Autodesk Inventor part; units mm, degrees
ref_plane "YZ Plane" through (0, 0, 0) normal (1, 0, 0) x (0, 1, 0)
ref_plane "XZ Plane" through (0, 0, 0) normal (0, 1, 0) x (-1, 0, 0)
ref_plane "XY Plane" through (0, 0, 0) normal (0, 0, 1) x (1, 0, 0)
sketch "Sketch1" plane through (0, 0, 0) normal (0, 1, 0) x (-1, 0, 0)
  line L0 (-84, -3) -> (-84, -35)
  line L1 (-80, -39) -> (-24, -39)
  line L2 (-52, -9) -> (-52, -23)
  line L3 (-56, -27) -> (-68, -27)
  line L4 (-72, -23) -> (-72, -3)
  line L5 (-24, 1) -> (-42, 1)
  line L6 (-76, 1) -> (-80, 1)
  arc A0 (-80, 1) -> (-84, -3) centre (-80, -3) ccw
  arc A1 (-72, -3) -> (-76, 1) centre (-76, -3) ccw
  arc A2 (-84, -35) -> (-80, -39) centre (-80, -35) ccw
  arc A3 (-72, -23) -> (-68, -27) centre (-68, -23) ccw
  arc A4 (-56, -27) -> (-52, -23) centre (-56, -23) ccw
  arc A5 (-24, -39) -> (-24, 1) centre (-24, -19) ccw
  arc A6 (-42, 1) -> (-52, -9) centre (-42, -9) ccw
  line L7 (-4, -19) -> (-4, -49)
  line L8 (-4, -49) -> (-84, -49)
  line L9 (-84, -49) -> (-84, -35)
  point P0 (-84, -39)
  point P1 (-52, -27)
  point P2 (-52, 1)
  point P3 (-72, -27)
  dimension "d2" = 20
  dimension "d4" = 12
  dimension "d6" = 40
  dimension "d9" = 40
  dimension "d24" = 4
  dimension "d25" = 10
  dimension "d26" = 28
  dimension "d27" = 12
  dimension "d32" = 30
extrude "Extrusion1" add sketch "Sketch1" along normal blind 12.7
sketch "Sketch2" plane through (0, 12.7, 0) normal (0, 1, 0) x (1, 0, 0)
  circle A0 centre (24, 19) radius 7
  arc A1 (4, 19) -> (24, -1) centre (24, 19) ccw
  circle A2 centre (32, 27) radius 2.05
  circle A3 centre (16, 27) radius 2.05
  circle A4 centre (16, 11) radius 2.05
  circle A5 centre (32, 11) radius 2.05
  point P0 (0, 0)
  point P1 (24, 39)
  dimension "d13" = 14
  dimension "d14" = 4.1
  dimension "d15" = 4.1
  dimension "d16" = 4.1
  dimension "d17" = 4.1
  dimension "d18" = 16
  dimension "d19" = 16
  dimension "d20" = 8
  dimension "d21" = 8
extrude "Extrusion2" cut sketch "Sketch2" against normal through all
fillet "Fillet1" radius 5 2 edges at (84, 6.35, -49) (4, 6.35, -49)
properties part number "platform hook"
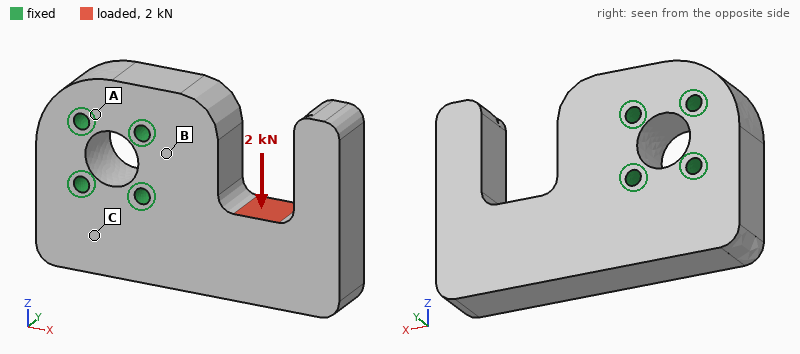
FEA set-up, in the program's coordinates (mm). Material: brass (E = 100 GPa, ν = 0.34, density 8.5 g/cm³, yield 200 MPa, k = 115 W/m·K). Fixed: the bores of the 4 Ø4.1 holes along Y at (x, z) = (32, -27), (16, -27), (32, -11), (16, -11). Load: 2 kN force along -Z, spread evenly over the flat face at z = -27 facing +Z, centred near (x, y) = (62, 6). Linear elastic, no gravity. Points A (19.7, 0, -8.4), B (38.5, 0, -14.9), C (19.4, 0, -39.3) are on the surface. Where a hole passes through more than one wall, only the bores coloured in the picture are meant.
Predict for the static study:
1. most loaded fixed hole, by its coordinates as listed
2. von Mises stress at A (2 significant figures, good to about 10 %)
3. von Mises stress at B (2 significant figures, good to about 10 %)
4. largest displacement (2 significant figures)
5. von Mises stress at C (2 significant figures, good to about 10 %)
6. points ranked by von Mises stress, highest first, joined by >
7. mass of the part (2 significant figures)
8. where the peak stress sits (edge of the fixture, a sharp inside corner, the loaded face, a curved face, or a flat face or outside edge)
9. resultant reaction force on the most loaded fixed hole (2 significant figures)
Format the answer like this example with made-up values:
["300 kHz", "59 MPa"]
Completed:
["(32, -11)", "4.1 MPa", "17 MPa", "26 µm", "7.9 MPa", "B > C > A", "340 g", "a curved face", "2.2 kN"]
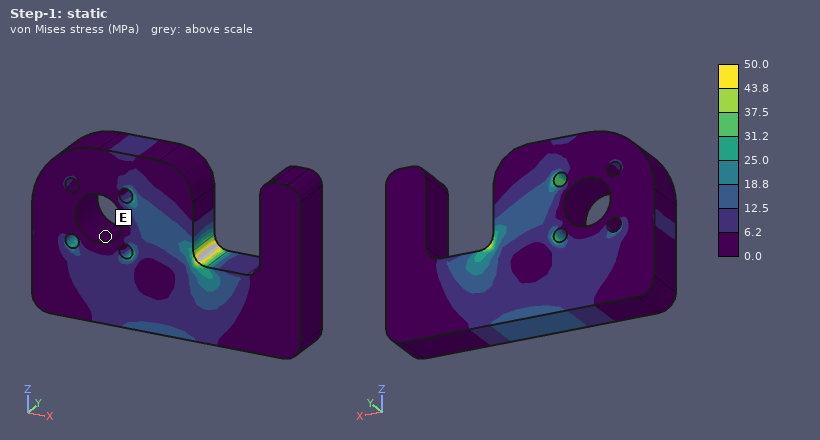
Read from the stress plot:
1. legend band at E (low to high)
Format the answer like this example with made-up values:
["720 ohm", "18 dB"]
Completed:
["0.0 to 6.2 MPa"]
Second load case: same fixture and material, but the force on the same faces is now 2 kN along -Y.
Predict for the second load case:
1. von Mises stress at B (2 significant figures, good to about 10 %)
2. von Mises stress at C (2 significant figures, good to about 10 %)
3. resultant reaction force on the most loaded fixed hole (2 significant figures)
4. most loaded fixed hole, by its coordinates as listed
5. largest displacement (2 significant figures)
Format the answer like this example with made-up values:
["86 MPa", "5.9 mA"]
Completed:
["39 MPa", "11 MPa", "2.3 kN", "(32, -27)", "0.12 mm"]
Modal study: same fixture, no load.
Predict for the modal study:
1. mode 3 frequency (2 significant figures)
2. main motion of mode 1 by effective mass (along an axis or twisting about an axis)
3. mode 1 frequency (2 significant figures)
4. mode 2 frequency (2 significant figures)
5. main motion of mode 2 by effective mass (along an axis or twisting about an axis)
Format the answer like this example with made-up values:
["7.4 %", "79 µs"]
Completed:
["3500 Hz", "along Y", "1900 Hz", "3300 Hz", "along Z"]
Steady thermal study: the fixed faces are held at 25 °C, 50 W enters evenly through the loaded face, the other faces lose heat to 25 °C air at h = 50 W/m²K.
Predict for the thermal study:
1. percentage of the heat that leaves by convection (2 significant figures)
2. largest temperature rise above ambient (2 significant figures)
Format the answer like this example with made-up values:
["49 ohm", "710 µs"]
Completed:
["15 %", "48 K"]
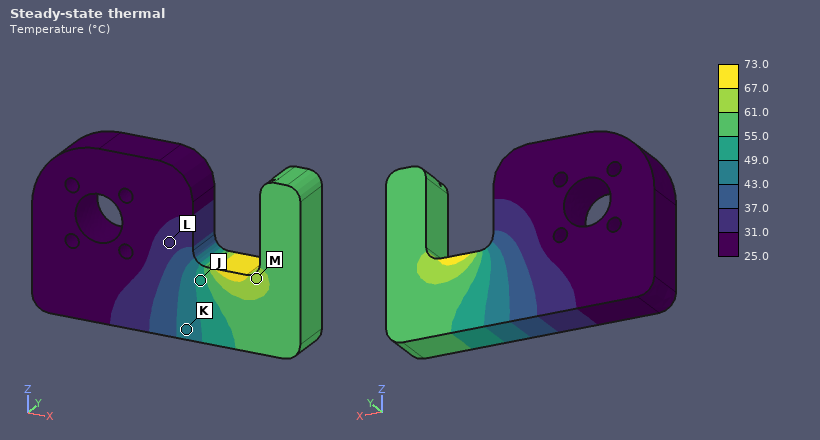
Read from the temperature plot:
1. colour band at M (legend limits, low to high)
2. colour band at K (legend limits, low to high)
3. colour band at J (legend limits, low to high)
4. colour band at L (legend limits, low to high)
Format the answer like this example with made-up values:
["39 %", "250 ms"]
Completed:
["61.0 to 67.0 °C", "43.0 to 49.0 °C", "49.0 to 55.0 °C", "31.0 to 37.0 °C"]
